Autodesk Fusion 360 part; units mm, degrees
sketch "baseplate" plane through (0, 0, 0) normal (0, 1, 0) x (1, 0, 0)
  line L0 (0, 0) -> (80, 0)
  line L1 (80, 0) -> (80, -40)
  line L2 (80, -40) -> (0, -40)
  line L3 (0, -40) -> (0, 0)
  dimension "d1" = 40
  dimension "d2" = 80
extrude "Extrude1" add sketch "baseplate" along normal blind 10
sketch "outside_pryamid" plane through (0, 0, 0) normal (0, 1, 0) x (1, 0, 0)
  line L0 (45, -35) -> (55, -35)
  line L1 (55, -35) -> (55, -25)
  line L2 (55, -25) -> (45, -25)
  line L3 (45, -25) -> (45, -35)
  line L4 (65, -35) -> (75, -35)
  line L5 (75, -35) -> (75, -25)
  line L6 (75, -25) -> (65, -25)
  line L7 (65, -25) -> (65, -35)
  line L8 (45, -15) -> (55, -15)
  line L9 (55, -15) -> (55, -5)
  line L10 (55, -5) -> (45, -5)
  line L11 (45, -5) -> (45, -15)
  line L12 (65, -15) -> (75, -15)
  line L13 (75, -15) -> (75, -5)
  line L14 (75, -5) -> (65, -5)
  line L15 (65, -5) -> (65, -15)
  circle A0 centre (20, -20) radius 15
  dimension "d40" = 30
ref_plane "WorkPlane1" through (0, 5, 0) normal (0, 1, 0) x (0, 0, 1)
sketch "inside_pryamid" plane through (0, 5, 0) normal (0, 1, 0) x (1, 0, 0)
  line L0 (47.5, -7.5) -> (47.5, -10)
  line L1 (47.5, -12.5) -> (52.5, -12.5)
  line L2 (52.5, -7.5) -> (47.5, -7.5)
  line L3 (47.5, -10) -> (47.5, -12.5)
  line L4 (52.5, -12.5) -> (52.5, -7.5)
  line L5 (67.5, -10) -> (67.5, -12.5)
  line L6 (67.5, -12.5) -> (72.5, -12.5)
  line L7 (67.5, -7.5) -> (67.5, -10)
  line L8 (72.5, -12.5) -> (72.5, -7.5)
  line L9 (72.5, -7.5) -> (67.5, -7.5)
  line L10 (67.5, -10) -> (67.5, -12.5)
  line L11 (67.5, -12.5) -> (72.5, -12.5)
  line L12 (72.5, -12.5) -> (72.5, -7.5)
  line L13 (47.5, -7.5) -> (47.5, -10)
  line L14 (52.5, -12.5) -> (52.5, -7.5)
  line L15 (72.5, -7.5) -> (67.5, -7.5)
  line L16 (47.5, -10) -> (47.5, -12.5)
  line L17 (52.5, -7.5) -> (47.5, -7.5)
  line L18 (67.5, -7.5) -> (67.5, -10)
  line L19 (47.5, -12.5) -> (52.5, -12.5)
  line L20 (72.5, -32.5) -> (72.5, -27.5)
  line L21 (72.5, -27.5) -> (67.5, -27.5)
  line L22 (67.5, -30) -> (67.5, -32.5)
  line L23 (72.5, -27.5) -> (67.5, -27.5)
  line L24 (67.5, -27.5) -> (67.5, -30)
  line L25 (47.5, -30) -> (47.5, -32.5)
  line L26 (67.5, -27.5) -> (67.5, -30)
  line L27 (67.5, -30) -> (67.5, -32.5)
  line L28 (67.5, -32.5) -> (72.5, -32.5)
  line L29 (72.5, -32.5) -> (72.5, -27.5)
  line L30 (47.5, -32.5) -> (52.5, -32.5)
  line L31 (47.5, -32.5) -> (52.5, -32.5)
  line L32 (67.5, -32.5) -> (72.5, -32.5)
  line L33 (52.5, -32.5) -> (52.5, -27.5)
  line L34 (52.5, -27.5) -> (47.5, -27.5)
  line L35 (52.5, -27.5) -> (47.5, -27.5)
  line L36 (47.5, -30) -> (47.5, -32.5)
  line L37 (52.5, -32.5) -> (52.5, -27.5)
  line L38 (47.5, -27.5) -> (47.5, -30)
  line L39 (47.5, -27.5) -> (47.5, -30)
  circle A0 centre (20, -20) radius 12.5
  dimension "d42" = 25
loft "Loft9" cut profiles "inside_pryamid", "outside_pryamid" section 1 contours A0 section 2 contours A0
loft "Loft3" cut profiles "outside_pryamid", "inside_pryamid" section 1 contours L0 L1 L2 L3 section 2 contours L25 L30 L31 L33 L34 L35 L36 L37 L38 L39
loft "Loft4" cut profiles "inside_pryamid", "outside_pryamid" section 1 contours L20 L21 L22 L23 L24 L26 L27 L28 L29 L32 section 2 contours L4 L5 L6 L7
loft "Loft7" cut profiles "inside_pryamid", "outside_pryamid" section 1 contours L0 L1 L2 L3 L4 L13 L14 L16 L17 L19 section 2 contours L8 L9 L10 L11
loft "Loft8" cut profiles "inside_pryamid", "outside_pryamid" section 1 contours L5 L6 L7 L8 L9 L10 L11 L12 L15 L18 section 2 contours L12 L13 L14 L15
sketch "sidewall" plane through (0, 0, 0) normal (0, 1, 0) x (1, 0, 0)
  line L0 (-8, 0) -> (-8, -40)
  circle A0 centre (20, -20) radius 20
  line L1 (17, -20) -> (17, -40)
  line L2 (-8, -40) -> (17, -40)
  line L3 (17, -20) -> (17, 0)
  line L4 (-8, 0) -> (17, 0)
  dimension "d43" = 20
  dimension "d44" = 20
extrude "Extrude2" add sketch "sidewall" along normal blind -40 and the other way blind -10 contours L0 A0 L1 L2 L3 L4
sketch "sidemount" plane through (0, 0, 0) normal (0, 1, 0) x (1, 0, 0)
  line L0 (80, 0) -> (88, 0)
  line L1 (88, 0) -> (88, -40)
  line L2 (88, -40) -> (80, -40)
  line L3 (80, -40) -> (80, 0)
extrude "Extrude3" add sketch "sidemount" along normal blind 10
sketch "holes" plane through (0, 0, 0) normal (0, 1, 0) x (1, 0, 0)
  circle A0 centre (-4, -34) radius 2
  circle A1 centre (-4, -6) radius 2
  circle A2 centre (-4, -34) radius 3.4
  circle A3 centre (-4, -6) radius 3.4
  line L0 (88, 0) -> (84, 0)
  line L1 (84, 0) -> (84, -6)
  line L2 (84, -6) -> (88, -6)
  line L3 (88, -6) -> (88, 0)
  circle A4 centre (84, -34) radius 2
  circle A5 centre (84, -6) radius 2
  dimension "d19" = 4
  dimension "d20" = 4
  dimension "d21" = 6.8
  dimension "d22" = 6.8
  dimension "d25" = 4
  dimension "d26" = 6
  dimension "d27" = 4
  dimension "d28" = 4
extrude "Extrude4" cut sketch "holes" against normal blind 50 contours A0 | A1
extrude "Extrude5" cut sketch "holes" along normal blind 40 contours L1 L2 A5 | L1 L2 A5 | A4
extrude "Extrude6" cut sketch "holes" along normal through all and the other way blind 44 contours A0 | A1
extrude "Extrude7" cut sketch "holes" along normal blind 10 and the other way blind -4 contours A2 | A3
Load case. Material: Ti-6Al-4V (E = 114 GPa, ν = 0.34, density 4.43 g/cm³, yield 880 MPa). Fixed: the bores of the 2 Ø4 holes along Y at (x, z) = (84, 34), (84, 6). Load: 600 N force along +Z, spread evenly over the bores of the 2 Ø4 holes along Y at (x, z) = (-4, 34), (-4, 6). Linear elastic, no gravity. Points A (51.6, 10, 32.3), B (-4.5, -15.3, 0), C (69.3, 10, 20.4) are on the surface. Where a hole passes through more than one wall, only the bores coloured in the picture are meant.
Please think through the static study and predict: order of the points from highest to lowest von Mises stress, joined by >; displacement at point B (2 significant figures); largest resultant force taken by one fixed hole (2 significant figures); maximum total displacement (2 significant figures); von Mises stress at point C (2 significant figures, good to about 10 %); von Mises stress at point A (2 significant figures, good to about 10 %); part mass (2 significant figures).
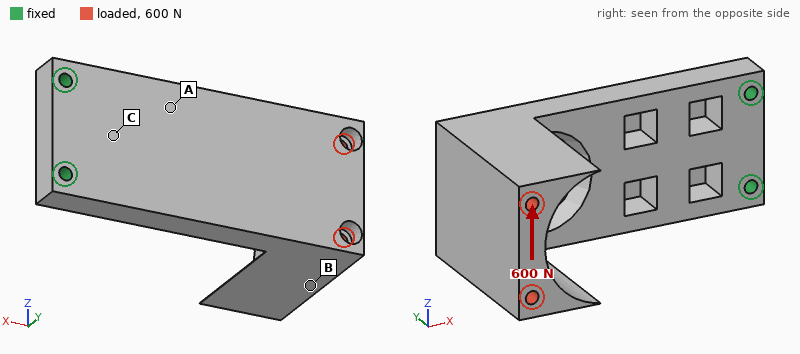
A > C > B
0.11 mm
1.9 kN
0.18 mm
13 MPa
22 MPa
230 g
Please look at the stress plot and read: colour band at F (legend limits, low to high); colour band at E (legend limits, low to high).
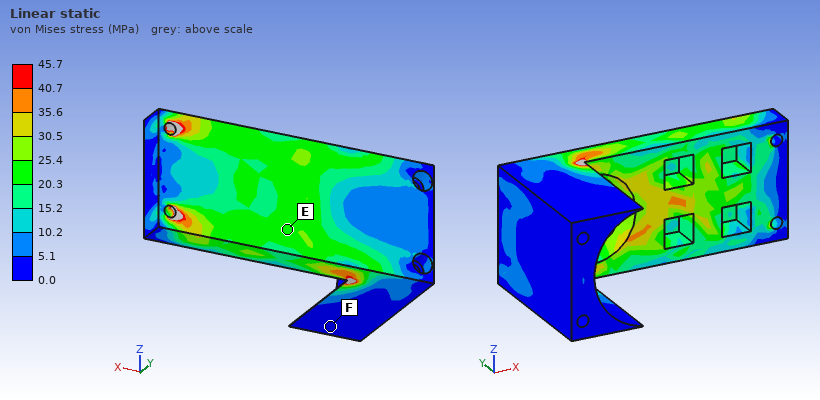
0.0 to 5.1 MPa
20.3 to 25.4 MPa
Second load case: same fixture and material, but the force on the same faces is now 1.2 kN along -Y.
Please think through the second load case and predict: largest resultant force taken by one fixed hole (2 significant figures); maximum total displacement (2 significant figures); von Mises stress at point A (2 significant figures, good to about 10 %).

630 N
1.3 mm
120 MPa
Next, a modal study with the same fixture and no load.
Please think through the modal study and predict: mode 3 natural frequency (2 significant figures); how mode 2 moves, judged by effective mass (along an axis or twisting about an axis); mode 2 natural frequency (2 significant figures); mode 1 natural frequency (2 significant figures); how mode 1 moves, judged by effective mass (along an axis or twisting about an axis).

2000 Hz
along Z
1100 Hz
490 Hz
along Y
